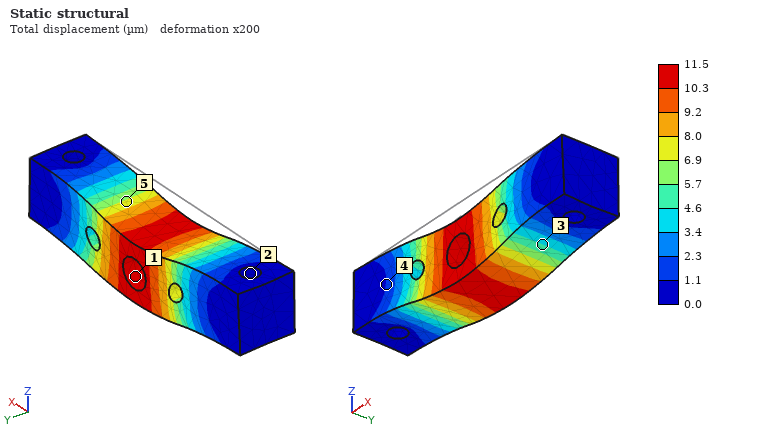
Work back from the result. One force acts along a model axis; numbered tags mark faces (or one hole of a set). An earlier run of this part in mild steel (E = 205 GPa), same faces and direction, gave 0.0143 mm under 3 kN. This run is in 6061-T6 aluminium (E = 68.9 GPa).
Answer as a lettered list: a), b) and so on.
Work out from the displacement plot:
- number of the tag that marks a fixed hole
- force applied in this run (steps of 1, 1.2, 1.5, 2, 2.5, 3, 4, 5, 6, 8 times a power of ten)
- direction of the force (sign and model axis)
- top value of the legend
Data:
a) 2
b) 800 N
c) -Z
d) 11.5 µm
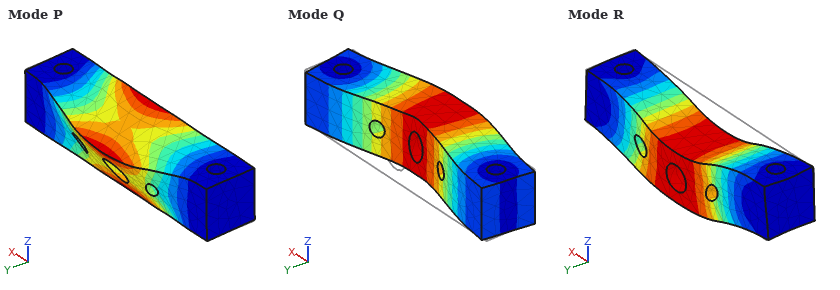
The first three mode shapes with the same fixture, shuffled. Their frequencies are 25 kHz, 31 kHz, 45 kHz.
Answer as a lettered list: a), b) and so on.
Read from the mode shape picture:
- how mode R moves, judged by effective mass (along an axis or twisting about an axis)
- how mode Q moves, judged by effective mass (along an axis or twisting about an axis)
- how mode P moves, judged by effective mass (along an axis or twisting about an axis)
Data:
a) along Z
b) along Y
c) twisting about X
